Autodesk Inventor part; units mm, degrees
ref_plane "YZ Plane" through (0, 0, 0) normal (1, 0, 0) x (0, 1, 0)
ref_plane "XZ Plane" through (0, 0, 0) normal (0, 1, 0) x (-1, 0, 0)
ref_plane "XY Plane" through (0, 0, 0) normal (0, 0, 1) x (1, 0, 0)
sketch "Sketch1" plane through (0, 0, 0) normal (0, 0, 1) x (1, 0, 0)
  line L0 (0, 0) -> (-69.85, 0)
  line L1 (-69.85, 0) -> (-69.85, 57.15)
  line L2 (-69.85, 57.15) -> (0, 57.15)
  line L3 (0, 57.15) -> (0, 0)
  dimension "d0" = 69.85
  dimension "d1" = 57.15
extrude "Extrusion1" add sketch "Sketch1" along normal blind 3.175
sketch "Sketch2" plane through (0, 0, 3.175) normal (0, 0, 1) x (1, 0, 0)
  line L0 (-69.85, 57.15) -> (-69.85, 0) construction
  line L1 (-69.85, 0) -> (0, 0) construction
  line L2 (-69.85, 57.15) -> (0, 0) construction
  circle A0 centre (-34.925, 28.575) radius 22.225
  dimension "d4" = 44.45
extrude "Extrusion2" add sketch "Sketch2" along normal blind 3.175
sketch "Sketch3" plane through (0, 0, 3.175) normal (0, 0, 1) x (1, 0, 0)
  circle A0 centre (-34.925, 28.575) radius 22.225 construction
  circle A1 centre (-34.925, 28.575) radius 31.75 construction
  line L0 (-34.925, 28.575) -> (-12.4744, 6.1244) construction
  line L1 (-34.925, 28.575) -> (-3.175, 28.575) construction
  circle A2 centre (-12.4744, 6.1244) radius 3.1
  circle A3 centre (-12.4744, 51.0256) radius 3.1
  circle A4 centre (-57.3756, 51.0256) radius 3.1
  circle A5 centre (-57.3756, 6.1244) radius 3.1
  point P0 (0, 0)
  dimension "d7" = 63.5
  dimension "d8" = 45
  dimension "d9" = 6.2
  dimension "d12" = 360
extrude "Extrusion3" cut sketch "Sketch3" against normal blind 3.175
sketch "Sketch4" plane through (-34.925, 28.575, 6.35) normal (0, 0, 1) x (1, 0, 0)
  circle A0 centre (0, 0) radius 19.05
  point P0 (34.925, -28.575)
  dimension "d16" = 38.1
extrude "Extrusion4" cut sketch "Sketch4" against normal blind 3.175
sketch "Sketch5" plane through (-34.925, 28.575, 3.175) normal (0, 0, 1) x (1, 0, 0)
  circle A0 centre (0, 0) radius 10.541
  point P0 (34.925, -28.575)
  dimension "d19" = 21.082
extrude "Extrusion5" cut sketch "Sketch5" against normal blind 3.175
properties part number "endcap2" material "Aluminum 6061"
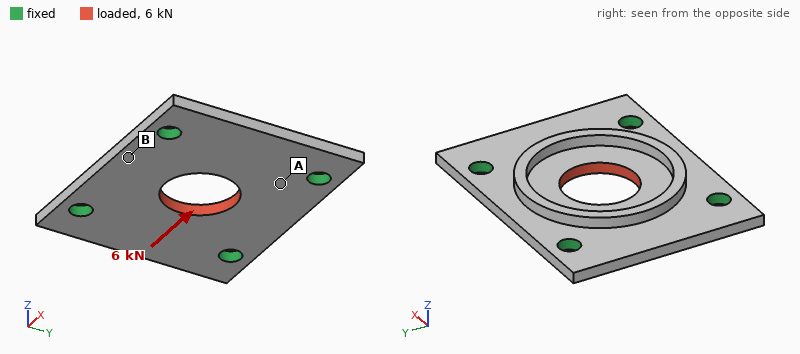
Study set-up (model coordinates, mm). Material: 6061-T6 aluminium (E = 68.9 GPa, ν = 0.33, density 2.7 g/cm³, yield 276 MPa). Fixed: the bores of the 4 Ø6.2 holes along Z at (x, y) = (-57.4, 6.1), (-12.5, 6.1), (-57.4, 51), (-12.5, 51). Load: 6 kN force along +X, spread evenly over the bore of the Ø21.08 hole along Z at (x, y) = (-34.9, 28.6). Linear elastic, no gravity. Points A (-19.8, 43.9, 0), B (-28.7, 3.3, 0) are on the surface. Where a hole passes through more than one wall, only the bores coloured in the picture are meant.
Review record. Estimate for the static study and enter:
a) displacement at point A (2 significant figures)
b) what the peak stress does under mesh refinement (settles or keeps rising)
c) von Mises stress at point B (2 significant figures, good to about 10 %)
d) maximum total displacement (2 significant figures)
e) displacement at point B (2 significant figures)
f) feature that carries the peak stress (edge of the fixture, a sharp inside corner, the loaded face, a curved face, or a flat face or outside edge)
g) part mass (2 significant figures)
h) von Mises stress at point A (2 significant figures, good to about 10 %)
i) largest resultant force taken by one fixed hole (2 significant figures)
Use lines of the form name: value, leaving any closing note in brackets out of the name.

displacement at point A: 5.2 µm
what the peak stress does under mesh refinement: keeps rising
von Mises stress at point B: 10.0 MPa
maximum total displacement: 14 µm
displacement at point B: 3.1 µm
feature that carries the peak stress: edge of the fixture
part mass: 34 g
von Mises stress at point A: 31 MPa
largest resultant force taken by one fixed hole: 1.6 kN
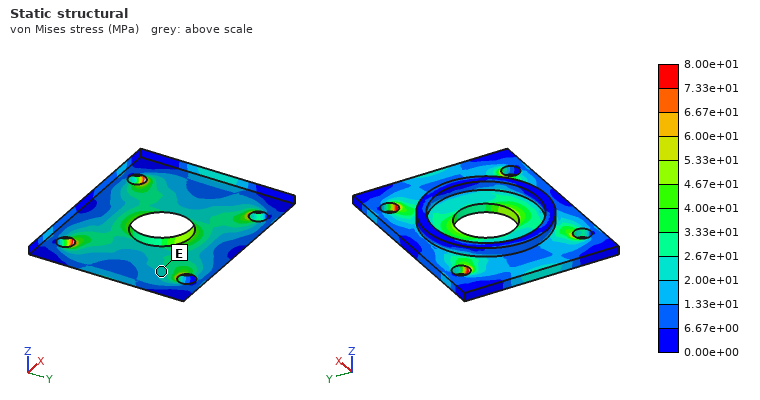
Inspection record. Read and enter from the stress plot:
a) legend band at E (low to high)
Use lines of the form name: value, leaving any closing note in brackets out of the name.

legend band at E: 2.00e+01 to 2.67e+01 MPa
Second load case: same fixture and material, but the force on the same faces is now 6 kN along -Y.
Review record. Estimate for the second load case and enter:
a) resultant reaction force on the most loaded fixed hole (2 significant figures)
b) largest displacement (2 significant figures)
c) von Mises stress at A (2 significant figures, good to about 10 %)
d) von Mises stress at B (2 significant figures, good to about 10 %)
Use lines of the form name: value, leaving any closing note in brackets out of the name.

resultant reaction force on the most loaded fixed hole: 1.6 kN
largest displacement: 16 µm
von Mises stress at A: 35 MPa
von Mises stress at B: 14 MPa
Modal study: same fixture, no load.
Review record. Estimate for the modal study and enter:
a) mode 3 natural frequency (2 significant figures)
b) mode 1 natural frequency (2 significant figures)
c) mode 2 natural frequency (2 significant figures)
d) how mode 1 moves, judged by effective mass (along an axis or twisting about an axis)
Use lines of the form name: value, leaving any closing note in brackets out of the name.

mode 3 natural frequency: 9400 Hz
mode 1 natural frequency: 8300 Hz
mode 2 natural frequency: 9400 Hz
how mode 1 moves, judged by effective mass: along Z
